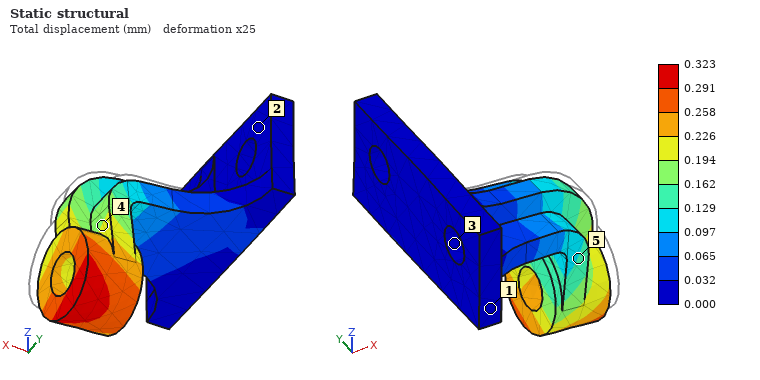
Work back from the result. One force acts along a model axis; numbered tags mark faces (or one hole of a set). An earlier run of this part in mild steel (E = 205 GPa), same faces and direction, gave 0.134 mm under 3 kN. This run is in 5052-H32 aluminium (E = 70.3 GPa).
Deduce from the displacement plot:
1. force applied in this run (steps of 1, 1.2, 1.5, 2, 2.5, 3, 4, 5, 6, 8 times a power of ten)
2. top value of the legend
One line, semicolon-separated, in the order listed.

2.5 kN; 0.323 mm
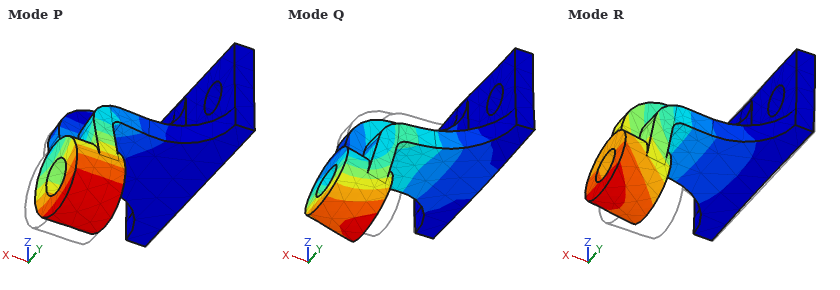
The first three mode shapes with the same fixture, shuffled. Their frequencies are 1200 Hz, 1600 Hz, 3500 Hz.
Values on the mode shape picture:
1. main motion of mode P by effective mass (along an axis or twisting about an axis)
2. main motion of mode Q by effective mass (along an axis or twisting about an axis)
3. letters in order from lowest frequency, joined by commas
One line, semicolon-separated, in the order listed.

along Y; along Z; R, P, Q
